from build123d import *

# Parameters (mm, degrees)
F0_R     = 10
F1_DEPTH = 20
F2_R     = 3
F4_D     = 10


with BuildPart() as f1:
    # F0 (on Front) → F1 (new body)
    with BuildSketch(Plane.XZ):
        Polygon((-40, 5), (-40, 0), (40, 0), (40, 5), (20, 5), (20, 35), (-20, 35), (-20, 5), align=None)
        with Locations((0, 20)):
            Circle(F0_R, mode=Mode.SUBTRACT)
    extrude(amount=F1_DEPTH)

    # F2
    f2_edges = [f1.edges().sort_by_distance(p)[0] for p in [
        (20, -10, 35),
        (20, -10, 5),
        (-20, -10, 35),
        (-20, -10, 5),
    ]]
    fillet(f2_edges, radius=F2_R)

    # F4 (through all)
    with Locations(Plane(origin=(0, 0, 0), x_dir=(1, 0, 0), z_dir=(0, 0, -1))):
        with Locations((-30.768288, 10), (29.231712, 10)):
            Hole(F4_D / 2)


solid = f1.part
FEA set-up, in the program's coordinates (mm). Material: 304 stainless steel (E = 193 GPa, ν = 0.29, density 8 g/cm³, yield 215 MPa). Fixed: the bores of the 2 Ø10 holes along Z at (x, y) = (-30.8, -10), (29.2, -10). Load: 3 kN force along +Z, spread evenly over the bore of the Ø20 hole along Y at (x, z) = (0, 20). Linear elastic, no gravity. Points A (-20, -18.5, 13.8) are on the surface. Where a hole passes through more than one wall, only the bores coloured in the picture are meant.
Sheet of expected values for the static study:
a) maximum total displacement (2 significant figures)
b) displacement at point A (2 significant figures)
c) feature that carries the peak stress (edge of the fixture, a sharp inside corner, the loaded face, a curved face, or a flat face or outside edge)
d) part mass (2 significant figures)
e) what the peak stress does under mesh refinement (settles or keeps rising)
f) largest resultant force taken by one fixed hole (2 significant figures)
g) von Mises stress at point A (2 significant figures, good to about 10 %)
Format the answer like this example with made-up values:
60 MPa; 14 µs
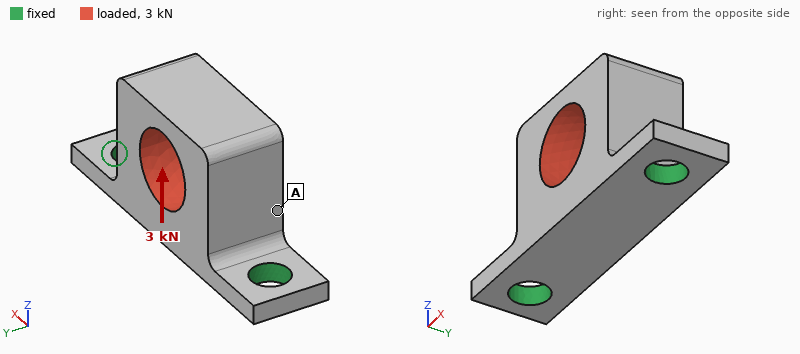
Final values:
5.7 µm; 4.8 µm; edge of the fixture; 200 g; keeps rising; 1.8 kN; 13 MPa
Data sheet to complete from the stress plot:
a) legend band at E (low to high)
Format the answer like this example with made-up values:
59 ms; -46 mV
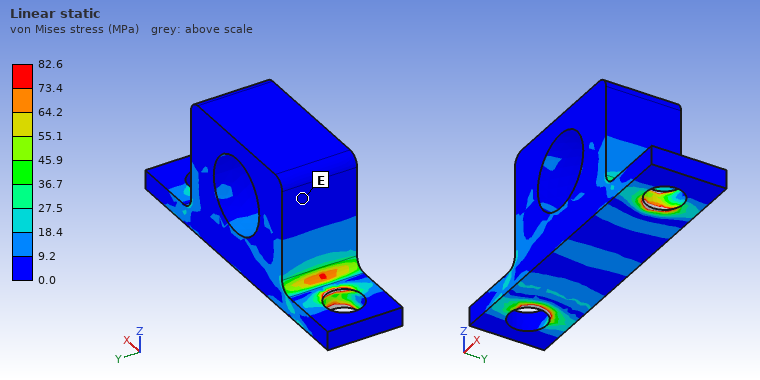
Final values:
0.0 to 9.2 MPa
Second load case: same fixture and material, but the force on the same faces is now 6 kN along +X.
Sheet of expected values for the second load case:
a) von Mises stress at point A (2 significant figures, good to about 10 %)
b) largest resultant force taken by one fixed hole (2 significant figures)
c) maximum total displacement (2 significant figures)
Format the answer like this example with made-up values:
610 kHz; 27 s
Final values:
24 MPa; 3.8 kN; 16 µm
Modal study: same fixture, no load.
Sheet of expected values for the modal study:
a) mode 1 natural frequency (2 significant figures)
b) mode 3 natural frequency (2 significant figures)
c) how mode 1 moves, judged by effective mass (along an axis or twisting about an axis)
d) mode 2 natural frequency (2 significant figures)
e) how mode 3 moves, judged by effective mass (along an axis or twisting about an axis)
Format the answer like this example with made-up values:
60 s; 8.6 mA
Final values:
3100 Hz; 9900 Hz; along Y; 8800 Hz; along Z
